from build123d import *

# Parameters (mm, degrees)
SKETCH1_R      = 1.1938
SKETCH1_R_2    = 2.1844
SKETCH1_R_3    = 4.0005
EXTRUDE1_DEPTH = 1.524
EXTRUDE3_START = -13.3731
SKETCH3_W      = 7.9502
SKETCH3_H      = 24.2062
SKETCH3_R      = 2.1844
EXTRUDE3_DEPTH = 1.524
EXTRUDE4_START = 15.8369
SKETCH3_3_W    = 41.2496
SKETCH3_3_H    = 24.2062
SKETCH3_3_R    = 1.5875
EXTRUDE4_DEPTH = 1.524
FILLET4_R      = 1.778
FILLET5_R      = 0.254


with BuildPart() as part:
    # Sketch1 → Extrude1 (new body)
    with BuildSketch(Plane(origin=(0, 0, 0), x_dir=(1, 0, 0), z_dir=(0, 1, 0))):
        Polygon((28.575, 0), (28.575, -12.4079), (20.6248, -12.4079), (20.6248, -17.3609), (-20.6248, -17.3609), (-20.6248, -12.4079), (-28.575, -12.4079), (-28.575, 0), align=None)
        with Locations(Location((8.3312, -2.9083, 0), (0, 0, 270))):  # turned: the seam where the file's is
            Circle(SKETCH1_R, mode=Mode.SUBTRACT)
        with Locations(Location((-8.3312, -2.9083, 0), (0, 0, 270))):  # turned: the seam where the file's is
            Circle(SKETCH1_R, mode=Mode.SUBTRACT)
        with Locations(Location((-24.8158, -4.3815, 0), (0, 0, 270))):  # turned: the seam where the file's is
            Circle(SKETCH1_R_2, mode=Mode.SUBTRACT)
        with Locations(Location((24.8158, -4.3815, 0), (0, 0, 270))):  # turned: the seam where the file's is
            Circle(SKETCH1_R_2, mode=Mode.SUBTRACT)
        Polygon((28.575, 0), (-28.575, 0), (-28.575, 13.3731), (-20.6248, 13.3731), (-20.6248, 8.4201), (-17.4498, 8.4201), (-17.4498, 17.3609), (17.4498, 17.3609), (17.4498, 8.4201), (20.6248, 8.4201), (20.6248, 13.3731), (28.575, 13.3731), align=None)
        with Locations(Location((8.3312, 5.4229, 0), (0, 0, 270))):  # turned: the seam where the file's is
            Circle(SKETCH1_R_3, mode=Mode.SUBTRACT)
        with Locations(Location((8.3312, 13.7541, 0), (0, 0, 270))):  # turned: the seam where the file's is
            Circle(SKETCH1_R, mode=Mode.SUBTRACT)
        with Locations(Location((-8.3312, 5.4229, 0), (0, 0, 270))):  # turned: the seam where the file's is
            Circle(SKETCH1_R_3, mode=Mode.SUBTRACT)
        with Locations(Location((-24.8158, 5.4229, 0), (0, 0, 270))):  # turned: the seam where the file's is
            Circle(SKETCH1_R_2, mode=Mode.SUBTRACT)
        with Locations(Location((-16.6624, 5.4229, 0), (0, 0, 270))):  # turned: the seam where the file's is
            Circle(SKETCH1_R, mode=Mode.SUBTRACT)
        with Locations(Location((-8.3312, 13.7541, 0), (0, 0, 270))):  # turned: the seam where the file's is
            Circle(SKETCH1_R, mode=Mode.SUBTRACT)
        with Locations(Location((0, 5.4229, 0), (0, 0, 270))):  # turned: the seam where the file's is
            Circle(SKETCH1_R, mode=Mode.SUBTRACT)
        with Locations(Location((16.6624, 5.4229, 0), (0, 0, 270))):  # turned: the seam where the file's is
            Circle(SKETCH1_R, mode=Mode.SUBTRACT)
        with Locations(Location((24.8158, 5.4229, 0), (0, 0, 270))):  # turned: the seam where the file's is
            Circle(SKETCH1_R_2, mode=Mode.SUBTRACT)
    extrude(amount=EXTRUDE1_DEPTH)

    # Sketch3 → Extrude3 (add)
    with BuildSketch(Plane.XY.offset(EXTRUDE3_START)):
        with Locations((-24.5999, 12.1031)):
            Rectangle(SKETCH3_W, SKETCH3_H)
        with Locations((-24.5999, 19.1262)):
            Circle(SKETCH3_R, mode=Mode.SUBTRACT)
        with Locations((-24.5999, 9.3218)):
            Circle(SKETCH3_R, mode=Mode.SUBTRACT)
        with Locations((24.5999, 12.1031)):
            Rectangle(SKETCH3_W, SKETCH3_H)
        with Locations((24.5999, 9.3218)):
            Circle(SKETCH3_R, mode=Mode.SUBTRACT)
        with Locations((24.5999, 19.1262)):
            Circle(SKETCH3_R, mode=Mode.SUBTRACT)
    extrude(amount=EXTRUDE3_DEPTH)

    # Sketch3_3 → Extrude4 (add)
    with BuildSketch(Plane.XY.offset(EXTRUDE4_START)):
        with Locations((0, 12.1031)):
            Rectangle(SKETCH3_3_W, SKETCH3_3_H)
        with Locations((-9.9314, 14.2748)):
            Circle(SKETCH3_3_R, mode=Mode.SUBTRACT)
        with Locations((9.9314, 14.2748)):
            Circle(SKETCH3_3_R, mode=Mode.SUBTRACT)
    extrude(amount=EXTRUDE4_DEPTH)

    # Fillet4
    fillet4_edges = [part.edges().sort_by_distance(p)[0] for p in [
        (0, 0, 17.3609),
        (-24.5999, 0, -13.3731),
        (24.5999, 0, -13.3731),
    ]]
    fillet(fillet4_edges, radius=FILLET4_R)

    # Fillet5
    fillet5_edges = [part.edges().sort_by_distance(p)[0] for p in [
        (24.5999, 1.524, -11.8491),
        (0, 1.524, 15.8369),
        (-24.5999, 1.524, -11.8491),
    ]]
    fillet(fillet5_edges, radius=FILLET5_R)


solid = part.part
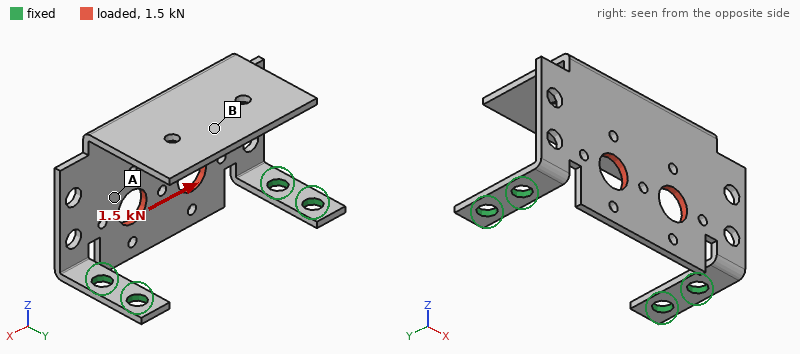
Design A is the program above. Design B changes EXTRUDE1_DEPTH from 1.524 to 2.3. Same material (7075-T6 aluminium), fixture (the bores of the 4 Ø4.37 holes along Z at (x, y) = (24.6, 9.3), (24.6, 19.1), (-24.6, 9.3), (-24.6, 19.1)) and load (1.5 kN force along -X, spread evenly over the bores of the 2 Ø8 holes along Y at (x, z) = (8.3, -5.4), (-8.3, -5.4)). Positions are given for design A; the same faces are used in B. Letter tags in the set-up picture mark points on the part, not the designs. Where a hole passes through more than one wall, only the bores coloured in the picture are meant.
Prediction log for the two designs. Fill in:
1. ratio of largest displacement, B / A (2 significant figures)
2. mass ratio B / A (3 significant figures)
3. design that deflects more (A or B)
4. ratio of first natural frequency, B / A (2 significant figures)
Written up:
0.61
1.28
A
1.3
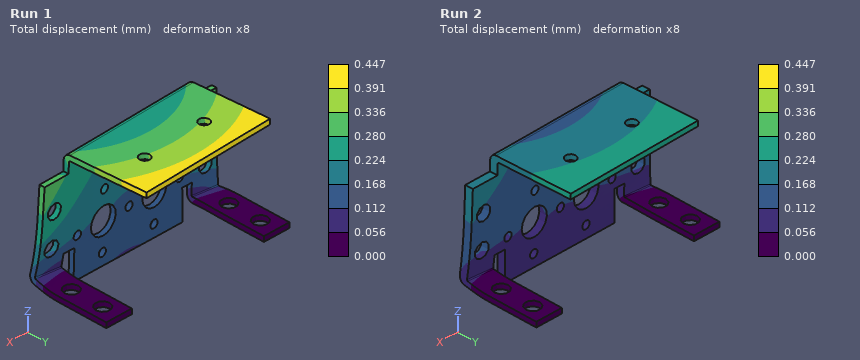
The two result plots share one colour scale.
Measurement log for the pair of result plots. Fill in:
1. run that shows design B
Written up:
Run 2
